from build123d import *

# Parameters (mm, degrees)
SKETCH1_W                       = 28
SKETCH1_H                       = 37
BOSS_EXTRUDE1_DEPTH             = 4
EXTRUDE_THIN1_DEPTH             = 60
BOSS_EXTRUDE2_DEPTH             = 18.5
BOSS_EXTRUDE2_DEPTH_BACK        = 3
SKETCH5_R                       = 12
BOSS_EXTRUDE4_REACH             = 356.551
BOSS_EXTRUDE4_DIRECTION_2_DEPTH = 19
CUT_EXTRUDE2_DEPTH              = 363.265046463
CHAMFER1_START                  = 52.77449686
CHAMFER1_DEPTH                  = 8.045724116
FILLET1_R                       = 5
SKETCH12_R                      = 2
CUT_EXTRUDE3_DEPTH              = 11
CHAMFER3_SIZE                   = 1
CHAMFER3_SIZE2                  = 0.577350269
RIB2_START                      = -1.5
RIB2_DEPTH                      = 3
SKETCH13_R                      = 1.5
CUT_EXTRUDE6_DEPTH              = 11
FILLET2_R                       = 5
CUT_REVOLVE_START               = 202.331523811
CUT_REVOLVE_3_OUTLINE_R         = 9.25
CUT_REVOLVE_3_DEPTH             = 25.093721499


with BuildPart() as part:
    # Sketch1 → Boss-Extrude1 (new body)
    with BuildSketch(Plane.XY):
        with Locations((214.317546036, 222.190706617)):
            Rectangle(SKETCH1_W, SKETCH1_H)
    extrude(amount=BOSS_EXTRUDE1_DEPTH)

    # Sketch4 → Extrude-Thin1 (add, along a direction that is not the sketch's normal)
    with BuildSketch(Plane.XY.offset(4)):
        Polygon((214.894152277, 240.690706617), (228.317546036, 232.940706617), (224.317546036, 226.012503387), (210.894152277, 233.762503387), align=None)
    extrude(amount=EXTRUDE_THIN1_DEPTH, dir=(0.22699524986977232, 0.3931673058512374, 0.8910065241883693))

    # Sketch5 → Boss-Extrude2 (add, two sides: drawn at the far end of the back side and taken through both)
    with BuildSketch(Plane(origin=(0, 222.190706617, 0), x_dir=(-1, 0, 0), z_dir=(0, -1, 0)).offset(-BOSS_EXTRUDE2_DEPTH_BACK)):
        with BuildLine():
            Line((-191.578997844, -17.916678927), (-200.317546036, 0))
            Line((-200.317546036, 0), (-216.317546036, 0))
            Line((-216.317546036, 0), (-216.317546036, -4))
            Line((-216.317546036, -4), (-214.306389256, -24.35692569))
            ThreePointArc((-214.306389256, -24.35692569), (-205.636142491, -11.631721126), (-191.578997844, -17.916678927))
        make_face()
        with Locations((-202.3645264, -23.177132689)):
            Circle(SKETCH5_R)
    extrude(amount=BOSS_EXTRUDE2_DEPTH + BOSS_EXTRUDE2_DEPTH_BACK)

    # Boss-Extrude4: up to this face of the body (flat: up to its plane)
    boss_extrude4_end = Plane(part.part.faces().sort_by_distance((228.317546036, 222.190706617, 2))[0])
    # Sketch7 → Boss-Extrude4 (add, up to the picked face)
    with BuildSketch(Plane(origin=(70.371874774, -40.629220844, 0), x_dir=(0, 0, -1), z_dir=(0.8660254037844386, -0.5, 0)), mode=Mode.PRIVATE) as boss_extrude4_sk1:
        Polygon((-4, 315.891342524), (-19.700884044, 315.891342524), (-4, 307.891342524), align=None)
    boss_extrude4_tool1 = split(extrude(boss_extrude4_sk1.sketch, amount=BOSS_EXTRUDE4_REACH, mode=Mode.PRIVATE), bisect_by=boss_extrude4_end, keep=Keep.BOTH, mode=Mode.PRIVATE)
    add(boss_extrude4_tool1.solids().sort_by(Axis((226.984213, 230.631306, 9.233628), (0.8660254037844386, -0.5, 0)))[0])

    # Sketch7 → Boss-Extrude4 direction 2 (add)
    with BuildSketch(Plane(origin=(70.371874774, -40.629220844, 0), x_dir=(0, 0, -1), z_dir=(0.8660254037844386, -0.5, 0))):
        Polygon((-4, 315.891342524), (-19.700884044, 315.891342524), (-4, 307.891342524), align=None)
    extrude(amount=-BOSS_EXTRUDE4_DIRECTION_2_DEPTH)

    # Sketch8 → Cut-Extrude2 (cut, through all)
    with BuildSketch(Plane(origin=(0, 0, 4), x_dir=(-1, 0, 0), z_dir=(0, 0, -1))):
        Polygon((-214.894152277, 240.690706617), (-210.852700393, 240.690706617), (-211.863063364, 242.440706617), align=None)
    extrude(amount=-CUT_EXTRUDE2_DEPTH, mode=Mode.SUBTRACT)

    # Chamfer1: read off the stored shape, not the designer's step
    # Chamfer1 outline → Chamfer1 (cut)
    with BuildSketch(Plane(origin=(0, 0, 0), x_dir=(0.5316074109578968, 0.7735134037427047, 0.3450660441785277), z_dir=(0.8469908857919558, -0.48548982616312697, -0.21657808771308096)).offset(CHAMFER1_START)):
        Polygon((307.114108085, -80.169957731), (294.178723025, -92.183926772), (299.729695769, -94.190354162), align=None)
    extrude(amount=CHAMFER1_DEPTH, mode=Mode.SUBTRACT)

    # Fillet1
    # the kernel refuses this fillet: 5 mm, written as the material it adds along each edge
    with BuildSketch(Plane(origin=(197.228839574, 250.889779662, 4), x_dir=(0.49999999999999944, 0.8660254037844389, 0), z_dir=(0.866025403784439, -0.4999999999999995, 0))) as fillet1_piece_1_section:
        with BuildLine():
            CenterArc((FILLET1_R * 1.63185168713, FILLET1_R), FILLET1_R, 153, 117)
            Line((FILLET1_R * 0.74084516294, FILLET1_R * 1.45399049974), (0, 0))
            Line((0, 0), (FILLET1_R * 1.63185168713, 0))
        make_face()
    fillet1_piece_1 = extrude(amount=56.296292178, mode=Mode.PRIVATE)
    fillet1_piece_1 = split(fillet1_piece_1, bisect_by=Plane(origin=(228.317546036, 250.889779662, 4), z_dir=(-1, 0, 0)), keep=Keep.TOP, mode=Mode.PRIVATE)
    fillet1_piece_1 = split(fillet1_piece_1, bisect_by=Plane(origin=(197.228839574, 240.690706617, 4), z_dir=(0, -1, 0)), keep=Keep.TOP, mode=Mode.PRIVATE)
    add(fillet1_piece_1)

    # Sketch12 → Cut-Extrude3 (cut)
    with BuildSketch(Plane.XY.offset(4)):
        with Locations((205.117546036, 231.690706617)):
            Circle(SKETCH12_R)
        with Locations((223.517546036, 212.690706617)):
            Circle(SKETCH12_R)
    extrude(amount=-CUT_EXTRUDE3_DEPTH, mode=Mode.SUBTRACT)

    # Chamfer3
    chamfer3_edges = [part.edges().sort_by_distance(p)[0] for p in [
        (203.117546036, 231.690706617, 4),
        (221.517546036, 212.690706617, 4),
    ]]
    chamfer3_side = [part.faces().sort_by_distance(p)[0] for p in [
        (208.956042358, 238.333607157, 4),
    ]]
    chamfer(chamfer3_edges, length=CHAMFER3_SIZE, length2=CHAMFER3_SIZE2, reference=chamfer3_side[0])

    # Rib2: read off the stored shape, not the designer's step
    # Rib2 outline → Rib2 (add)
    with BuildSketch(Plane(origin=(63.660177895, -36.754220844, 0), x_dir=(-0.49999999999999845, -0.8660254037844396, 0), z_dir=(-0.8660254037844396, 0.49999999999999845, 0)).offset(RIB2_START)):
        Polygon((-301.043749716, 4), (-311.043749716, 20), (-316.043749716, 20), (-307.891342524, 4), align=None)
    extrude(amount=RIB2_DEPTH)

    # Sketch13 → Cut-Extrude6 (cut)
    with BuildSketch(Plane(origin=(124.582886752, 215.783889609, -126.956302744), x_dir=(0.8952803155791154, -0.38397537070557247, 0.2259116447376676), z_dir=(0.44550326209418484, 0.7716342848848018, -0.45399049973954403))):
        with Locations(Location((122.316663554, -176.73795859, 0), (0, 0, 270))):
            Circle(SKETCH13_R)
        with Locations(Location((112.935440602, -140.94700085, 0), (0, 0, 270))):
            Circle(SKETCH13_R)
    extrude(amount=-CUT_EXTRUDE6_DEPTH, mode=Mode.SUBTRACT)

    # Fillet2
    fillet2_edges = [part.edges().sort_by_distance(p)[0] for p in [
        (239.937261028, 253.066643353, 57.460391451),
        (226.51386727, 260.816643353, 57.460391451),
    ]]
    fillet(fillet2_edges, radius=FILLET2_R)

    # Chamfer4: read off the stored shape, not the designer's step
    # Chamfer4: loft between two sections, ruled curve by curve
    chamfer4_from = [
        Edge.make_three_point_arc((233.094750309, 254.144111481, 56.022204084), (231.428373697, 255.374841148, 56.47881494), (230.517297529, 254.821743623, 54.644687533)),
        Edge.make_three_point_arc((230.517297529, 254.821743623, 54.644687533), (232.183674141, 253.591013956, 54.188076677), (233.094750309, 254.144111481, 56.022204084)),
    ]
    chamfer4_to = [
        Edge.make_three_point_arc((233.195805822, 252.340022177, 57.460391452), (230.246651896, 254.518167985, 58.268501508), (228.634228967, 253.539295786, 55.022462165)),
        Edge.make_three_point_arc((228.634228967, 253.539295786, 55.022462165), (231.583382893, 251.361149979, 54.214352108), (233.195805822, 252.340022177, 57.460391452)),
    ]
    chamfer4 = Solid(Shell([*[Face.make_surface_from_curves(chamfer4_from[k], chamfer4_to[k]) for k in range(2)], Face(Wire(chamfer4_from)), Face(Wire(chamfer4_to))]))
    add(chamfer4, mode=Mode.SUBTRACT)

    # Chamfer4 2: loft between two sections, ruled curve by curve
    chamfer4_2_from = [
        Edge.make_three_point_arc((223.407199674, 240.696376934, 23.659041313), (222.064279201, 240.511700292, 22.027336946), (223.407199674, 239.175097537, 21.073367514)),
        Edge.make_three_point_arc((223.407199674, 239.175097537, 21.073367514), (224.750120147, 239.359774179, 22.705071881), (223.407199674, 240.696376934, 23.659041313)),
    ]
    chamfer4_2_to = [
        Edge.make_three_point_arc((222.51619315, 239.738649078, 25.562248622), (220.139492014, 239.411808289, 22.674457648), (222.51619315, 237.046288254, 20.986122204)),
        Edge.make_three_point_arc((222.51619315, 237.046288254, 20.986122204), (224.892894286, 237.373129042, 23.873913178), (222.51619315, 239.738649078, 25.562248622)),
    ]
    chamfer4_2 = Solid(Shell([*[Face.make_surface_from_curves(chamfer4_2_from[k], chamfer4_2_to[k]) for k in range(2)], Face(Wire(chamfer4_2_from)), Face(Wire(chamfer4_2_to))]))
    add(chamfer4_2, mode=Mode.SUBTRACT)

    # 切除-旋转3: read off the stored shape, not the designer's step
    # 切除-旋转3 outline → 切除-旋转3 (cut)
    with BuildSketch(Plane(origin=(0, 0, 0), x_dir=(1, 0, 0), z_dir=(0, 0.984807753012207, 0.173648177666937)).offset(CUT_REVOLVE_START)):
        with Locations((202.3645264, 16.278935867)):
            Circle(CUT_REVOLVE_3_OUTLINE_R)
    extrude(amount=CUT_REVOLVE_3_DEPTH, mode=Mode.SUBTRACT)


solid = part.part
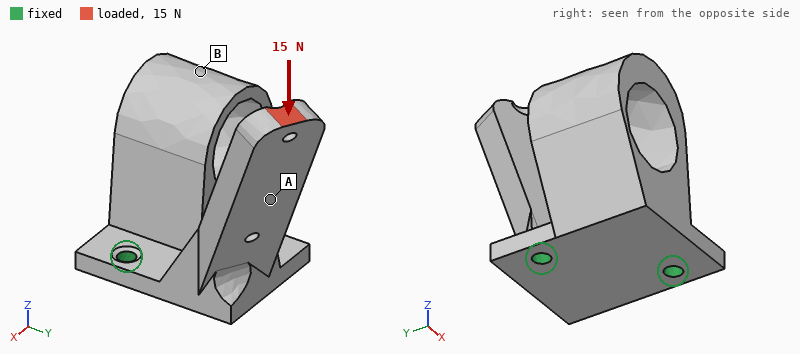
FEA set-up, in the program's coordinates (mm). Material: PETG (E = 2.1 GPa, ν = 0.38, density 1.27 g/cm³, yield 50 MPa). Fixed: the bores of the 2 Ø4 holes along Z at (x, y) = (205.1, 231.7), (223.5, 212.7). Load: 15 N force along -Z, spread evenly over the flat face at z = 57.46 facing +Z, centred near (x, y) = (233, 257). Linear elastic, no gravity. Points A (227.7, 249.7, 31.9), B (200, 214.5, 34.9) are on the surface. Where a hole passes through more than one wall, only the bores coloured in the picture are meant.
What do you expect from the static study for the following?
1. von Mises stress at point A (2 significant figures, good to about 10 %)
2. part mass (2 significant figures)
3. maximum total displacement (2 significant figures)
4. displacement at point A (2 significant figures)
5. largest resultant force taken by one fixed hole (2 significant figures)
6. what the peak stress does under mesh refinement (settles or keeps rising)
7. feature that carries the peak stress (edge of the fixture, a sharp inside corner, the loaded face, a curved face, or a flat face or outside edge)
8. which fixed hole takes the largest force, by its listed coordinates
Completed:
1.6 MPa
24 g
1.0 mm
0.49 mm
15 N
keeps rising
edge of the fixture
(205.1, 231.7)
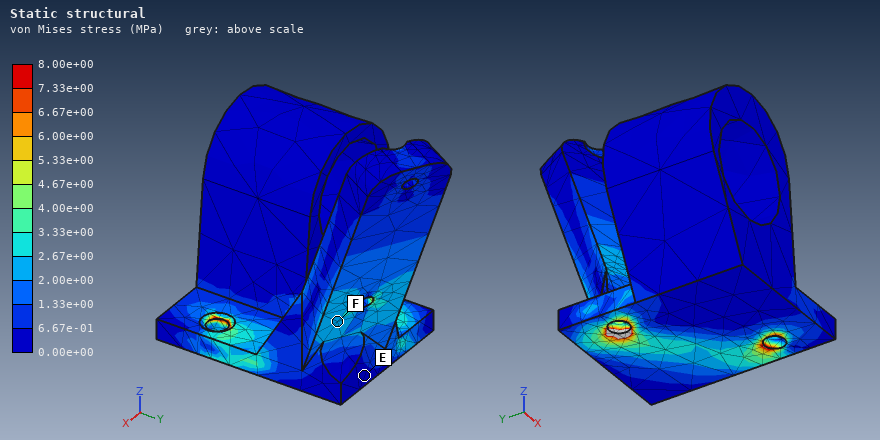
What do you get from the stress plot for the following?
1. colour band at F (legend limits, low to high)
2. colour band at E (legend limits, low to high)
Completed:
2.00e+00 to 2.67e+00 MPa
0.00e+00 to 6.67e-01 MPa
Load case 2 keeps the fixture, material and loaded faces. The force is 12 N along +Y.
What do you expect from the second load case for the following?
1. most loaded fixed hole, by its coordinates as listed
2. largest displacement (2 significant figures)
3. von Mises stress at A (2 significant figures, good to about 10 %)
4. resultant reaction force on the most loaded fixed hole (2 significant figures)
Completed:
(223.5, 212.7)
1.1 mm
1.9 MPa
22 N
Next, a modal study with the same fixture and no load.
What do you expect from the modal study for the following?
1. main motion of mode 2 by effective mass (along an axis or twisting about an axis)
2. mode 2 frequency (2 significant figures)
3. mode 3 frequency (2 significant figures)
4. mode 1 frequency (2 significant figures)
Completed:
along X
580 Hz
720 Hz
280 Hz
